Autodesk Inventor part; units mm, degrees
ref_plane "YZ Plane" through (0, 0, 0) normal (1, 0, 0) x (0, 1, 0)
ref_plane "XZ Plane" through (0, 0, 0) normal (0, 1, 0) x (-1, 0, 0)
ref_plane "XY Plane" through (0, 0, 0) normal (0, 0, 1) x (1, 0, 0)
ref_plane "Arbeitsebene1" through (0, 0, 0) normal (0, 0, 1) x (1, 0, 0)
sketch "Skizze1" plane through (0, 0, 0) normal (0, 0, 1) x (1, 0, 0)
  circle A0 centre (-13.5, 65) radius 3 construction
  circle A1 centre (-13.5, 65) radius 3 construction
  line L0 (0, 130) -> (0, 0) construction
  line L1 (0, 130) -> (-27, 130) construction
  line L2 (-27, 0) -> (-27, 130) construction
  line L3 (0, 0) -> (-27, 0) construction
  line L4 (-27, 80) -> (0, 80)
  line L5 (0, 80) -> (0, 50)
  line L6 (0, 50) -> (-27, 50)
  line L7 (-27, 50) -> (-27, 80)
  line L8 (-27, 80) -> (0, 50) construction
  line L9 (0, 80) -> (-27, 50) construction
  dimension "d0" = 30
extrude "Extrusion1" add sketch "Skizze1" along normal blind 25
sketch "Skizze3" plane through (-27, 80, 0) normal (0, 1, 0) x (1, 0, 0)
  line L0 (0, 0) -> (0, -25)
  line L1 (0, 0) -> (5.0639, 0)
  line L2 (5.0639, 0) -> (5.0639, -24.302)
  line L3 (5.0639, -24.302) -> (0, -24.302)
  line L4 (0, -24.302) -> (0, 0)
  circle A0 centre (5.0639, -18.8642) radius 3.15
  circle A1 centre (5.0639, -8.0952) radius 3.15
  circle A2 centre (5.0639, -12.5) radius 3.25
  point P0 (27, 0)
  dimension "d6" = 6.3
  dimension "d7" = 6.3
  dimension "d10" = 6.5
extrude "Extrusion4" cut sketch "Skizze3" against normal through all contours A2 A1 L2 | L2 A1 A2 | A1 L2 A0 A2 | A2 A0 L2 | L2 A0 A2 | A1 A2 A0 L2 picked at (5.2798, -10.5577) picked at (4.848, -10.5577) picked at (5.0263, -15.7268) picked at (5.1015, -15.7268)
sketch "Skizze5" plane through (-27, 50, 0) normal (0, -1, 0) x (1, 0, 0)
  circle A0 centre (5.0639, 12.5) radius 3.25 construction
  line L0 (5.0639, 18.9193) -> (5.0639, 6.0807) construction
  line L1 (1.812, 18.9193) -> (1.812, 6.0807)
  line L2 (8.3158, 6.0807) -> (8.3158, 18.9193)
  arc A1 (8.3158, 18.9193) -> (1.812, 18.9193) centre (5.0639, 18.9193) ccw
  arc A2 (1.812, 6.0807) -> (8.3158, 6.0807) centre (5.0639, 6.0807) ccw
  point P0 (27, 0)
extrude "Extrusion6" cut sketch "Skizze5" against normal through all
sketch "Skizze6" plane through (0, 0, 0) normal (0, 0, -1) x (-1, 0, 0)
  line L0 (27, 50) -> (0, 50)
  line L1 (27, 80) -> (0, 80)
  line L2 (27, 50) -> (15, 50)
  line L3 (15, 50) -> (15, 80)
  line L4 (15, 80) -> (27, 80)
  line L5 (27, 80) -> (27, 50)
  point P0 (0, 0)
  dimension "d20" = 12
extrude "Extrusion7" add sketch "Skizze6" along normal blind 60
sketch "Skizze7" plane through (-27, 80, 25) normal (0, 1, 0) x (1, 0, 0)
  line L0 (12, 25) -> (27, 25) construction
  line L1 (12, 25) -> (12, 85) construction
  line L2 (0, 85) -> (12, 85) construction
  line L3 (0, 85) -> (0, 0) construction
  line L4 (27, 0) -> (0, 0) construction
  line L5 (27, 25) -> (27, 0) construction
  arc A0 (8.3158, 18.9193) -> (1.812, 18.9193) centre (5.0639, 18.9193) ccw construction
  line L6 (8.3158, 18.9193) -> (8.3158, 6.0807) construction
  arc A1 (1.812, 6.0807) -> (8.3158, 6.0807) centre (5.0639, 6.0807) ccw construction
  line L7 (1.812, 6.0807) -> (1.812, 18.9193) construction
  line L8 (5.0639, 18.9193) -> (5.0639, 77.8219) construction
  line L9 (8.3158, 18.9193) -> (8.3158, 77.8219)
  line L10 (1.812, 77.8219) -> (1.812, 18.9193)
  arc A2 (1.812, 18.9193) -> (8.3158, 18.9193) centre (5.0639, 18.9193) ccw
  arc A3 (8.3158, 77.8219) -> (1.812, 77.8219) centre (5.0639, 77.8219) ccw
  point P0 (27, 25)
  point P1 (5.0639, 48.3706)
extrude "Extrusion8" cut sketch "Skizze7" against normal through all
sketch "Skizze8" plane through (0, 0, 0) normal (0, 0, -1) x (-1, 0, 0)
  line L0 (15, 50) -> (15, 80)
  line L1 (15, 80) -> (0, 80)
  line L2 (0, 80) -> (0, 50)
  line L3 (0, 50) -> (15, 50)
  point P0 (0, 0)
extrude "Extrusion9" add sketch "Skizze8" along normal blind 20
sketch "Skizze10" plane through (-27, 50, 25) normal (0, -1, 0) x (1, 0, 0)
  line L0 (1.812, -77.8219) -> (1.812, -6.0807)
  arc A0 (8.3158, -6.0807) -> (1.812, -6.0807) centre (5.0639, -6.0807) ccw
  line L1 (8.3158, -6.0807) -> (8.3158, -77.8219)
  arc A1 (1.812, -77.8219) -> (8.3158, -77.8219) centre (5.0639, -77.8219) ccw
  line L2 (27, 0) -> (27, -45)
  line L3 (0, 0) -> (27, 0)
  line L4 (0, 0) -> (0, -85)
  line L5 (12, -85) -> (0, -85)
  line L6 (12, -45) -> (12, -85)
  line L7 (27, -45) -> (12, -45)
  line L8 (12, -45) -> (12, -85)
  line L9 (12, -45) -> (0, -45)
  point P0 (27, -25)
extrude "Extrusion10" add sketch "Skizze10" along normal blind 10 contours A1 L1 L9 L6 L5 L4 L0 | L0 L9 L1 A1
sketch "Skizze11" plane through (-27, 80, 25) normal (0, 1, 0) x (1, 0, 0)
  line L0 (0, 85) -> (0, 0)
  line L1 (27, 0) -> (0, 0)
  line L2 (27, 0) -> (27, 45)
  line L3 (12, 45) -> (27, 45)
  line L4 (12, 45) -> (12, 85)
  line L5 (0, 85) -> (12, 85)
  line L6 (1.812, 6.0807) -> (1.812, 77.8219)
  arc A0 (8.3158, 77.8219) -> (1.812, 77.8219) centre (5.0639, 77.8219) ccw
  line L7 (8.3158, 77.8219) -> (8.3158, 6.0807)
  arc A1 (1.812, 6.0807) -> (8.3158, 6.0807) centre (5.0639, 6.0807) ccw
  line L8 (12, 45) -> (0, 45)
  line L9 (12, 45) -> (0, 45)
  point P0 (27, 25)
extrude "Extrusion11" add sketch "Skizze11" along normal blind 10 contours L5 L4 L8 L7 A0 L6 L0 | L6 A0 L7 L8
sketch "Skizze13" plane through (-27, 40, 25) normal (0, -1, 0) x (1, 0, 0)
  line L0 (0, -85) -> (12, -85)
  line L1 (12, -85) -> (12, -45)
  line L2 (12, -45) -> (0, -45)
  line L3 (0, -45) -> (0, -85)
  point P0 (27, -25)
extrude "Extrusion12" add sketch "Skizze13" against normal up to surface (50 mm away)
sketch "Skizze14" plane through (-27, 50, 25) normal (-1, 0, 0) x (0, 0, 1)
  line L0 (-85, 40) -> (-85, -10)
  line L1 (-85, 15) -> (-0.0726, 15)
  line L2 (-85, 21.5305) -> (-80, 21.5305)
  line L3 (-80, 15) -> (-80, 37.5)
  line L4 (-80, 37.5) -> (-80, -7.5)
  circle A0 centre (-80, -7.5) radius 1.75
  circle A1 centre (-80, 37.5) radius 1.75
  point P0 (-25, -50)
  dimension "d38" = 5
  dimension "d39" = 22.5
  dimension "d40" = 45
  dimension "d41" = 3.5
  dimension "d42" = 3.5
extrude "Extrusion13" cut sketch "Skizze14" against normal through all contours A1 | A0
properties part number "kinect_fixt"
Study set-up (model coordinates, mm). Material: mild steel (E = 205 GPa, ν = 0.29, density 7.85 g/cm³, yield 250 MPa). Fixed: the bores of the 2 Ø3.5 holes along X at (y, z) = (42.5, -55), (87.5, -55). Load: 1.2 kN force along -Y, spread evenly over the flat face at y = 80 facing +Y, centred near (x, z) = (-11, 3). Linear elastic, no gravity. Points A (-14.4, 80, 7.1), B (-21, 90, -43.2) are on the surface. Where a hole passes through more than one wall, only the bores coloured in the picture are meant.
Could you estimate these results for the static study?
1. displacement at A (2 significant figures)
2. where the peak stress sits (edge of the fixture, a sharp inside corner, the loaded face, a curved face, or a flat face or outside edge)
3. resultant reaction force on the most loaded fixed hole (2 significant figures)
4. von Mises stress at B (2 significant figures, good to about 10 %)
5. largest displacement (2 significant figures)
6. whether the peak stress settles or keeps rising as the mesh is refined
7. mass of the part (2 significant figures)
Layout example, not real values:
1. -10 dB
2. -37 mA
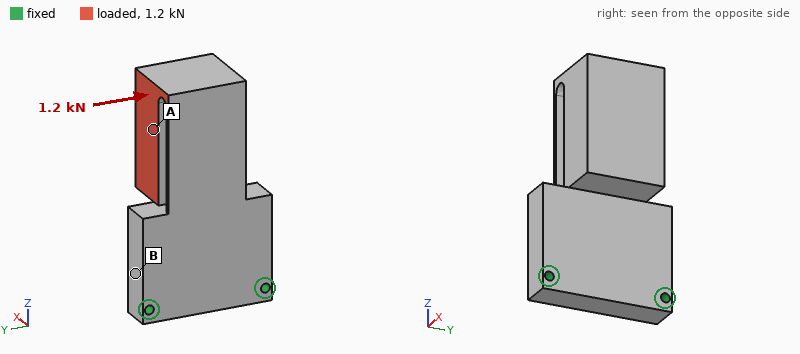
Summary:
1. 9.8 µm
2. edge of the fixture
3. 1.7 kN
4. 15 MPa
5. 15 µm
6. keeps rising
7. 410 g
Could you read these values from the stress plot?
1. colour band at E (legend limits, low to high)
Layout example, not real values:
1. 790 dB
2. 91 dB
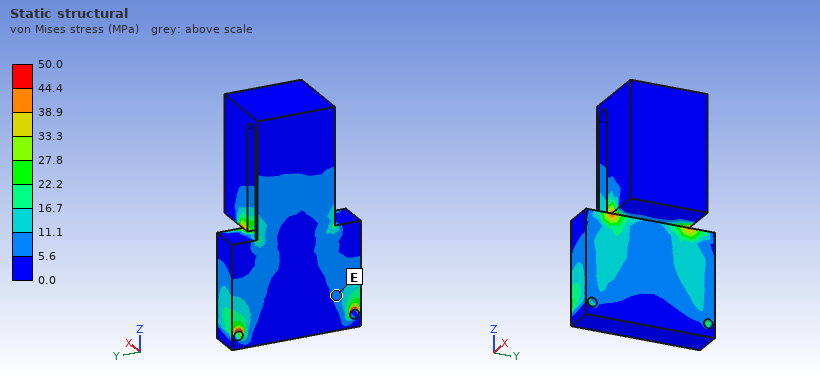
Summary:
1. 5.6 to 11.1 MPa
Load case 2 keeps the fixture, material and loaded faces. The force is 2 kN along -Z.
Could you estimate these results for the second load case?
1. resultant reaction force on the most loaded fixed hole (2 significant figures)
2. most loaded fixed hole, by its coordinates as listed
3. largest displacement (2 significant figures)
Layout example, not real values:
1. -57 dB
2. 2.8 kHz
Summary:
1. 1.7 kN
2. (87.5, -55)
3. 92 µm
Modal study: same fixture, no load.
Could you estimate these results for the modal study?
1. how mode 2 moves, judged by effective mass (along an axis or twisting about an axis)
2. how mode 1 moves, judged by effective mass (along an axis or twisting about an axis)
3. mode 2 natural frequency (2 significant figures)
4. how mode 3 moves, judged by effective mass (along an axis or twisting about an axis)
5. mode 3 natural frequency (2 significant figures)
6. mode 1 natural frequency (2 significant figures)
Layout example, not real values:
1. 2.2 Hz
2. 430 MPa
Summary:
1. along Y
2. along X
3. 3600 Hz
4. along X
5. 4800 Hz
6. 920 Hz
